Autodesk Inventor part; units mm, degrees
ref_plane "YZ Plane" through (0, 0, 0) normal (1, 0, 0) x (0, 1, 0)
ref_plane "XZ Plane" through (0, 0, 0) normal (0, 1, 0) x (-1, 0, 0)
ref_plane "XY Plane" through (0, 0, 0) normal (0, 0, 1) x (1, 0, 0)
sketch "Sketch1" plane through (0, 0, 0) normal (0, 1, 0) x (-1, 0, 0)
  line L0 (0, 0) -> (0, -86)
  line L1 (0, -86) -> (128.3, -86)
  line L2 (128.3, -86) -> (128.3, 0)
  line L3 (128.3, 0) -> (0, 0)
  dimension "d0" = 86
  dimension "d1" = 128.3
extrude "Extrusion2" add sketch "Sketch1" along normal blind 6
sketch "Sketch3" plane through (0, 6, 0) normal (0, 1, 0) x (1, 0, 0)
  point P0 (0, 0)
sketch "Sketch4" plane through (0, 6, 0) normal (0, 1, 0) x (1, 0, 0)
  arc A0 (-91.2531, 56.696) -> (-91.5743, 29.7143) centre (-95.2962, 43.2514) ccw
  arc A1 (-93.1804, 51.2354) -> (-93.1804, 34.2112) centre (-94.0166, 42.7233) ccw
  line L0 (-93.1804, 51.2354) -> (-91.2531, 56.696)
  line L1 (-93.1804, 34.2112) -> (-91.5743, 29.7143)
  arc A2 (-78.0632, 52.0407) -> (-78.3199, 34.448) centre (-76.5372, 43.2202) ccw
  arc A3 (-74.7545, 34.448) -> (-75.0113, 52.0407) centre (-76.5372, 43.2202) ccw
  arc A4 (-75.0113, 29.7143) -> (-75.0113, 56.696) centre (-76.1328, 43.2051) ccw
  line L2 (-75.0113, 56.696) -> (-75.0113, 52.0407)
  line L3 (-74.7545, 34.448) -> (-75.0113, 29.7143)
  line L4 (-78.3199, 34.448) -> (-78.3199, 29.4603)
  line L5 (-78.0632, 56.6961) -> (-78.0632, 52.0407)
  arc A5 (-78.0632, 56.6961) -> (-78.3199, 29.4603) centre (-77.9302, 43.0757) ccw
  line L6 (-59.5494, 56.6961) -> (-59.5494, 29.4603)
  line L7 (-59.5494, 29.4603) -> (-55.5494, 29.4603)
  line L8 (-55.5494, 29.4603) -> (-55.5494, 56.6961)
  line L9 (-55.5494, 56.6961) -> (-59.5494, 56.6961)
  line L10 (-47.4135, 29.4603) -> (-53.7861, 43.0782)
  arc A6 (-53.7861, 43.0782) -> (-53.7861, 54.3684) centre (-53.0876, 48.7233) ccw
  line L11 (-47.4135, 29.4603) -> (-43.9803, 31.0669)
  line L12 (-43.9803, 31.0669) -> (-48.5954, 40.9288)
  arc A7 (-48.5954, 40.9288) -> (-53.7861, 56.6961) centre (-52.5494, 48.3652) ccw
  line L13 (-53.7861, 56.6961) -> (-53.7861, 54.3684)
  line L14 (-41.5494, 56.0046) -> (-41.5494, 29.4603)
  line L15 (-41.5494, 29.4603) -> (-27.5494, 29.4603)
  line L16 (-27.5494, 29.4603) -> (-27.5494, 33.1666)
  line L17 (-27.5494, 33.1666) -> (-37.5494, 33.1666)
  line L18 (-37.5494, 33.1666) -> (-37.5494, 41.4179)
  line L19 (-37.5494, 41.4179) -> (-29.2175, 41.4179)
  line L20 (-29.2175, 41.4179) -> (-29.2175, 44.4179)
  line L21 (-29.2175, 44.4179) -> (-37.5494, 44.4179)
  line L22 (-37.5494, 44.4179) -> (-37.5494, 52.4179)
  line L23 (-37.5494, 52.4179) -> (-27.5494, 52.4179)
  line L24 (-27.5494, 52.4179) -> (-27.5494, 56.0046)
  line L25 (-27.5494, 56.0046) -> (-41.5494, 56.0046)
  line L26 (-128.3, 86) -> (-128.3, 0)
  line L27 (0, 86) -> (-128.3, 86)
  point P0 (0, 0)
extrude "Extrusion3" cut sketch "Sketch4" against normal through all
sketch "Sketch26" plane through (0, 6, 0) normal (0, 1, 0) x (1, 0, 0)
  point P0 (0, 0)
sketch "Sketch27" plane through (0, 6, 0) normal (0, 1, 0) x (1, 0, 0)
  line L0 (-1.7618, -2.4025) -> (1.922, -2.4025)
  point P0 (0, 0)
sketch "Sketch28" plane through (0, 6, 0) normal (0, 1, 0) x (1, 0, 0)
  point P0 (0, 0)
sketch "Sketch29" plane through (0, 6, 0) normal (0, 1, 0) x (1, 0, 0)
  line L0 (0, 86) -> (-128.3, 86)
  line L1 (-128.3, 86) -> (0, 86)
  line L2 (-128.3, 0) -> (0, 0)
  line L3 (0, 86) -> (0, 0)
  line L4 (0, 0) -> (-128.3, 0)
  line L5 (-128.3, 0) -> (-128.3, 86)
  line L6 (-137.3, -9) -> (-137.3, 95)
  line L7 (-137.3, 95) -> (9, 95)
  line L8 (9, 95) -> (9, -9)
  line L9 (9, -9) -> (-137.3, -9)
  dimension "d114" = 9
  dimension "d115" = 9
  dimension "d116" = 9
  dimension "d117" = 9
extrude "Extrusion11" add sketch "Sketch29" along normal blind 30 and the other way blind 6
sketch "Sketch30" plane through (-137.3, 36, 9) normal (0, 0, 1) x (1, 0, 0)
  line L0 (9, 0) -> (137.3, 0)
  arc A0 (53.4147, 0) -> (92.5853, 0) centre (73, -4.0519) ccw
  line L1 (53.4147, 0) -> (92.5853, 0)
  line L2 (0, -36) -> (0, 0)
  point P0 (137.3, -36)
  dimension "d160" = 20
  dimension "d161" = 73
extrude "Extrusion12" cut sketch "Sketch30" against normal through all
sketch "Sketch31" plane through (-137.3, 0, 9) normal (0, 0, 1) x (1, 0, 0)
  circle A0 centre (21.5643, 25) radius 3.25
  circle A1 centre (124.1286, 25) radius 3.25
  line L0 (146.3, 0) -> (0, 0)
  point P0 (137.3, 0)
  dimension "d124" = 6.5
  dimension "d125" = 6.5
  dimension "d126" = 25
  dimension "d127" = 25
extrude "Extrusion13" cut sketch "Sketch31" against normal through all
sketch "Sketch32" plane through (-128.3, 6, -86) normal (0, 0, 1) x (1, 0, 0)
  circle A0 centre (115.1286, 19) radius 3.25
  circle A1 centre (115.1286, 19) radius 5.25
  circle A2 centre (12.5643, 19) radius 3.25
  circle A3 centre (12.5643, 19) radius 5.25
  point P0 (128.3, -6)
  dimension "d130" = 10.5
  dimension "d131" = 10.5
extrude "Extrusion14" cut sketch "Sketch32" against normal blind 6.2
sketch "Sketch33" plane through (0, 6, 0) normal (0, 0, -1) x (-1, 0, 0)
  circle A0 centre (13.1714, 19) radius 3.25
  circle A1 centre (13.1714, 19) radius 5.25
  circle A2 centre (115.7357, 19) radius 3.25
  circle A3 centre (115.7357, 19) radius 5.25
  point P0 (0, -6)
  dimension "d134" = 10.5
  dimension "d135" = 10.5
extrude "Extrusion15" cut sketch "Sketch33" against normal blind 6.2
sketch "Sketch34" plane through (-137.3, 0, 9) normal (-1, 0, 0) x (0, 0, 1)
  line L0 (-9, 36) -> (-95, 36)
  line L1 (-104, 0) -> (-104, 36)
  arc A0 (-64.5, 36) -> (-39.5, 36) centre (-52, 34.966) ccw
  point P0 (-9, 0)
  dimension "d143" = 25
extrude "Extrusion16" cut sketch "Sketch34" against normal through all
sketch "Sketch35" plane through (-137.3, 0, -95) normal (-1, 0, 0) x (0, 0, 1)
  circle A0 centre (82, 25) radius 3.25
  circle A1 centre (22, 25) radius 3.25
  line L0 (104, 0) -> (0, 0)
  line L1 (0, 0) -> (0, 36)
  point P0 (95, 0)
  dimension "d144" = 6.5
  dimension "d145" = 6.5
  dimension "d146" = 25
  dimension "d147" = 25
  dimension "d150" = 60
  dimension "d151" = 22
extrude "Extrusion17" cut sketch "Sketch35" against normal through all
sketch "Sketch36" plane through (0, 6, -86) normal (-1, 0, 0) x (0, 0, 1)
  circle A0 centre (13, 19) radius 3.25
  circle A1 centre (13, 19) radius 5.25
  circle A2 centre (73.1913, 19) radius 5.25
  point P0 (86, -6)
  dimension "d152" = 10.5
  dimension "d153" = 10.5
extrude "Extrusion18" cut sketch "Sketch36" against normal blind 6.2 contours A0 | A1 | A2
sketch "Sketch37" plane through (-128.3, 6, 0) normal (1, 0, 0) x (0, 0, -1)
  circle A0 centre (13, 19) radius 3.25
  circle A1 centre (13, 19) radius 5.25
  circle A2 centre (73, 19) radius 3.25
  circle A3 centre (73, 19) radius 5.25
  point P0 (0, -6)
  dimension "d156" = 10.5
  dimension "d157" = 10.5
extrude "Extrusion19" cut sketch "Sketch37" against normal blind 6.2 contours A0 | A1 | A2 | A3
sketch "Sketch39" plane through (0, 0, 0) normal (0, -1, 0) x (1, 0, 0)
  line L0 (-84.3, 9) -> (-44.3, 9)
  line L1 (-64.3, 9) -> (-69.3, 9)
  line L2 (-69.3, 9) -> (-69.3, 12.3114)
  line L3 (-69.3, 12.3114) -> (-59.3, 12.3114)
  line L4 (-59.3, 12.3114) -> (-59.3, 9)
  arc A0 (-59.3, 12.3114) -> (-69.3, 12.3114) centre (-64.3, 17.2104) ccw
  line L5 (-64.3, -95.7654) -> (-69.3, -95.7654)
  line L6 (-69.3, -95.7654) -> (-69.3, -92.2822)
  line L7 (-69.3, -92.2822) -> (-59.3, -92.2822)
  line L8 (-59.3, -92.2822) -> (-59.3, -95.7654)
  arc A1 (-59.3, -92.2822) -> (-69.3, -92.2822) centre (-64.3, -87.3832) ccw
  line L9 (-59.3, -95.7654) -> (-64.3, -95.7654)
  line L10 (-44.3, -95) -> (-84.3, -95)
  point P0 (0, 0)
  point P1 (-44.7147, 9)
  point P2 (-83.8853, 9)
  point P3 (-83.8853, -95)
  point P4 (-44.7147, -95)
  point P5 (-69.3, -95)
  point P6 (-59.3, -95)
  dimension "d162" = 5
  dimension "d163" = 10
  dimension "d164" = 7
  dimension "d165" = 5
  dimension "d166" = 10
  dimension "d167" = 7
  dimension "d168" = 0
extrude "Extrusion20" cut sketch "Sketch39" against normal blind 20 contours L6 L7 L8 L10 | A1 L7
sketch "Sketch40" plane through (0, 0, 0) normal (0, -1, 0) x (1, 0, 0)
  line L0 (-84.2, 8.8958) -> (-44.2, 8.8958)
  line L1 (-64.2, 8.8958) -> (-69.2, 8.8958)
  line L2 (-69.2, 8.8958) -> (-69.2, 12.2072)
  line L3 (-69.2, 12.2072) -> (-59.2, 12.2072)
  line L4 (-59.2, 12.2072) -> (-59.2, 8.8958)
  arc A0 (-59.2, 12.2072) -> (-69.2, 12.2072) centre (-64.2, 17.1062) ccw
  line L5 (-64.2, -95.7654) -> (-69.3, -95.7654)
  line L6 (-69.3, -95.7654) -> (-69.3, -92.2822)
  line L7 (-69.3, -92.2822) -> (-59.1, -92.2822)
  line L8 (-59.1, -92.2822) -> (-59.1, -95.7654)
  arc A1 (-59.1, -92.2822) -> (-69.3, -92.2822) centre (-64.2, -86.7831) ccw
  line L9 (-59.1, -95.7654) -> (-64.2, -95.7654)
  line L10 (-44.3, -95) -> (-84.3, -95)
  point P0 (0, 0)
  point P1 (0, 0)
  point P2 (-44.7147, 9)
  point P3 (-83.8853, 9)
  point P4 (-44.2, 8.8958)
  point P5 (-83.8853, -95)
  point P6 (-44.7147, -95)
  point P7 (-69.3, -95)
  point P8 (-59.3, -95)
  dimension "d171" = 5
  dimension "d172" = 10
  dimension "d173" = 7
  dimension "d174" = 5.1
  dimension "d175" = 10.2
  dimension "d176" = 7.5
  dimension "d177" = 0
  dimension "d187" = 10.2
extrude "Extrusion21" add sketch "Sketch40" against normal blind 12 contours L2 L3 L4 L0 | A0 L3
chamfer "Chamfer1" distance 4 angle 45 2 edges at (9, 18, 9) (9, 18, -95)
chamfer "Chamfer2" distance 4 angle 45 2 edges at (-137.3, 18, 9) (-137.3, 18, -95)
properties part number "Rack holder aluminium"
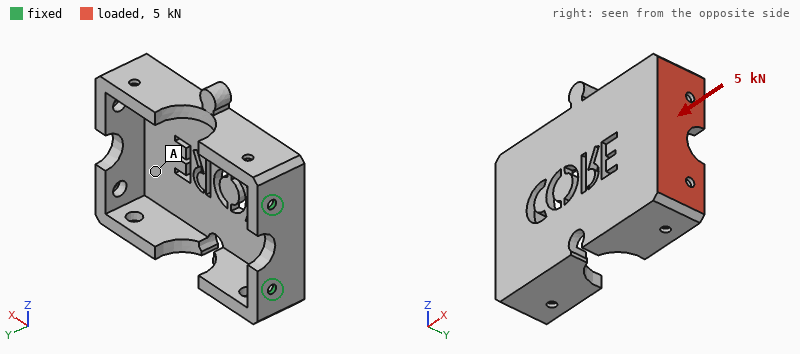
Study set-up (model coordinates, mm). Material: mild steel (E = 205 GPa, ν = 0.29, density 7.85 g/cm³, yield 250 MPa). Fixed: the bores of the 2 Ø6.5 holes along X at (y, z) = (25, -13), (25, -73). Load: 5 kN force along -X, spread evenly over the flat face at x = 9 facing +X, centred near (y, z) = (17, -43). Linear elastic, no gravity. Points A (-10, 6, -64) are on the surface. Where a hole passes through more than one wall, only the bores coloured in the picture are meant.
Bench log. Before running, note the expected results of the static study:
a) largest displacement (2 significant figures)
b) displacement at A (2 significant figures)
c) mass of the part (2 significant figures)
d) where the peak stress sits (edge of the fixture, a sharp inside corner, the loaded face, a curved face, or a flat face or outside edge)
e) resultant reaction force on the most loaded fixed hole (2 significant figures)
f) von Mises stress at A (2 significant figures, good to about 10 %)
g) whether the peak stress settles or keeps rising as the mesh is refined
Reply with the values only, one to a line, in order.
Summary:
0.28 mm
0.12 mm
1.5 kg
edge of the fixture
2.5 kN
22 MPa
keeps rising
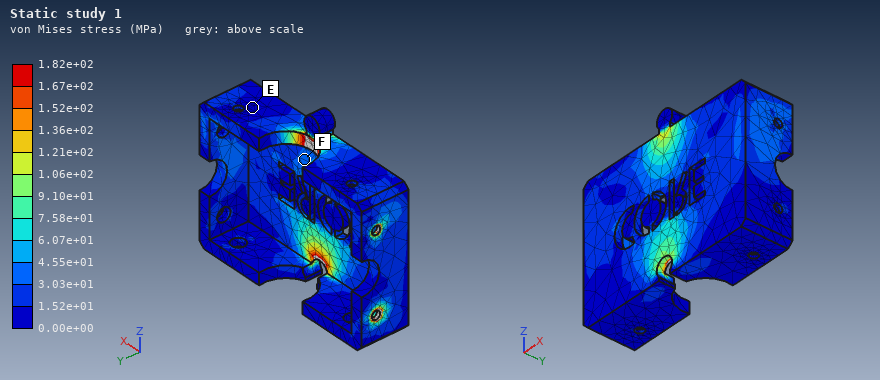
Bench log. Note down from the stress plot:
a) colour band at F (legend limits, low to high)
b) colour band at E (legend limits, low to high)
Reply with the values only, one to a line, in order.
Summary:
3.03e+01 to 4.55e+01 MPa
0.00e+00 to 1.52e+01 MPa
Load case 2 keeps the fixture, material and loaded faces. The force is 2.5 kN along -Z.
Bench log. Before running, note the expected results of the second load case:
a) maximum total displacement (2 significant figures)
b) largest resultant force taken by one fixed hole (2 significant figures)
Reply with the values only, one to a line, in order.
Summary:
0.71 mm
5.7 kN
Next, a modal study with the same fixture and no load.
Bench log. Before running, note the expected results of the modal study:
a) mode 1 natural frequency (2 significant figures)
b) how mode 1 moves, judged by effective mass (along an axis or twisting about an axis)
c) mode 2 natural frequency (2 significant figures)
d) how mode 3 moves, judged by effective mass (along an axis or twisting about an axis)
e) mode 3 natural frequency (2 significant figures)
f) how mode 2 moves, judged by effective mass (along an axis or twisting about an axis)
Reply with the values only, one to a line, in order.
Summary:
190 Hz
along Y
430 Hz
along X
900 Hz
along Z
